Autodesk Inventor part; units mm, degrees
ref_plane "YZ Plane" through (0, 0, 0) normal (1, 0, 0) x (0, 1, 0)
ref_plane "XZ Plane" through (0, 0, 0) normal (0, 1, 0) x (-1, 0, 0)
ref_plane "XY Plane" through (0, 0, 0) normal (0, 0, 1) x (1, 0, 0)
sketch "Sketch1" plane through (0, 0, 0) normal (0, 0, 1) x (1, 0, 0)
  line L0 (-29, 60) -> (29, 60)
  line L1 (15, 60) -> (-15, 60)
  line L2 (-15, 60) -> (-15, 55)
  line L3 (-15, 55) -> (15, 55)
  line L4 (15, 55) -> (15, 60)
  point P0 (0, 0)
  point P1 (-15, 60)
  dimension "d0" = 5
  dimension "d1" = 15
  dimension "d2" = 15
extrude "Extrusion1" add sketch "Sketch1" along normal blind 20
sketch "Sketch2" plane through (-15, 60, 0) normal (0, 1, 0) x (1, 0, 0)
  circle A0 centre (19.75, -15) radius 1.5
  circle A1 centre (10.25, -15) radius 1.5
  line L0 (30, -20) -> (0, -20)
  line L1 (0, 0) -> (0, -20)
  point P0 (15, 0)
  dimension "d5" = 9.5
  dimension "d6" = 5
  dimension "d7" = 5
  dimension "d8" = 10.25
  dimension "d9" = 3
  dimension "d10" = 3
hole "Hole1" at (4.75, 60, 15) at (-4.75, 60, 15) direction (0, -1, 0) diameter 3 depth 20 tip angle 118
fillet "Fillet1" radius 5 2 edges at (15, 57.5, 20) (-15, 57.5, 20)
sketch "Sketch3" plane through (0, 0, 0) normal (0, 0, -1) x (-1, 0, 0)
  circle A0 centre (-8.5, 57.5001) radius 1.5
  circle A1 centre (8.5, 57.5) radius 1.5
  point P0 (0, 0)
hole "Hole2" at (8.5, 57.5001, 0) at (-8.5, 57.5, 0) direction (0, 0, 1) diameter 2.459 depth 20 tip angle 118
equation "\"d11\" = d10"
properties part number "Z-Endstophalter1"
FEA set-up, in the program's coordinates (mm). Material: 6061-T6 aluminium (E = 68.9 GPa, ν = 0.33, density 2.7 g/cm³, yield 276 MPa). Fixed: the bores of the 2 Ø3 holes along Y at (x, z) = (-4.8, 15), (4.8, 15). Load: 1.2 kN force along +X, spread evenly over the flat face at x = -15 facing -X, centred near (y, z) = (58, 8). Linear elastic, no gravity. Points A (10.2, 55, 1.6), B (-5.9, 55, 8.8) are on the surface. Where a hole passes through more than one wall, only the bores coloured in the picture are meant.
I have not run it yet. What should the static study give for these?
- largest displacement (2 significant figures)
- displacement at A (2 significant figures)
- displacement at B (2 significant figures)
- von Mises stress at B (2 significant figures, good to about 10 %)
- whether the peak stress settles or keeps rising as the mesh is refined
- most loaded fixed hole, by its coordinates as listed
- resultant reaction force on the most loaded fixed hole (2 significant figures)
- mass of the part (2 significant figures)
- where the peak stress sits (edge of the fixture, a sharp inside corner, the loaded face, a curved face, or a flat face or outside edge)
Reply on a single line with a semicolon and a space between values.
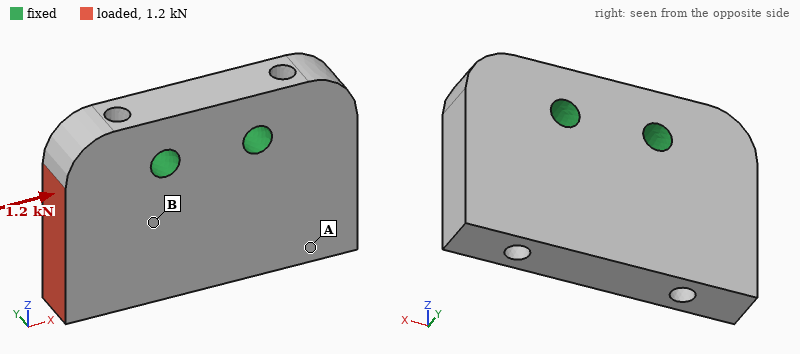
15 µm; 7.5 µm; 4.9 µm; 27 MPa; keeps rising; (-4.8, 15); 1.0 kN; 7.3 g; edge of the fixture
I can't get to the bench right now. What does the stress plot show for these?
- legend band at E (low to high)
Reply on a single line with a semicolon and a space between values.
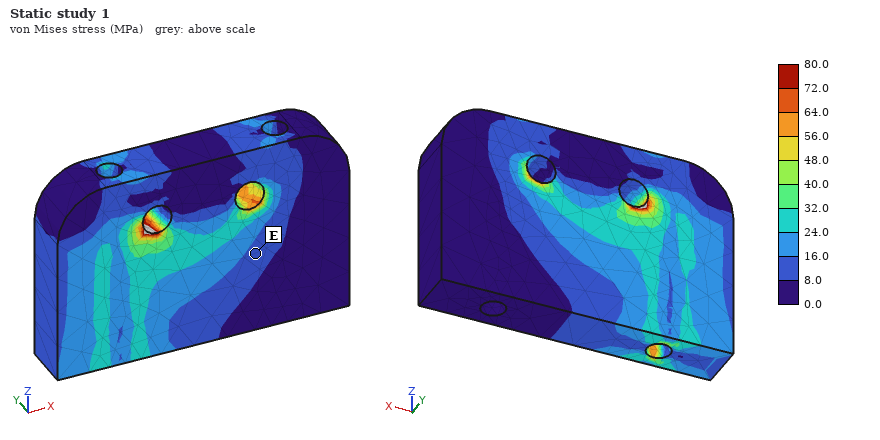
8.0 to 16.0 MPa
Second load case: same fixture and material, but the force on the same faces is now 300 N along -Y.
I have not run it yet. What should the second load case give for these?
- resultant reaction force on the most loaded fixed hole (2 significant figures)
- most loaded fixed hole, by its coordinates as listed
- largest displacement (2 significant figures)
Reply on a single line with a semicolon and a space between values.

410 N; (-4.8, 15); 33 µm
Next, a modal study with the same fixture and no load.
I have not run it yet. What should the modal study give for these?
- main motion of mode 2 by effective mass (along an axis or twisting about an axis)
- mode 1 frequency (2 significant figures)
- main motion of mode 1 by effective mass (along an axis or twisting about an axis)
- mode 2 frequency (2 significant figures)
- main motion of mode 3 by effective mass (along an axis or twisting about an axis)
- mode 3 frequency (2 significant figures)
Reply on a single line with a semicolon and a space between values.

twisting about Z; 15 kHz; along Y; 18 kHz; along X; 25 kHz
